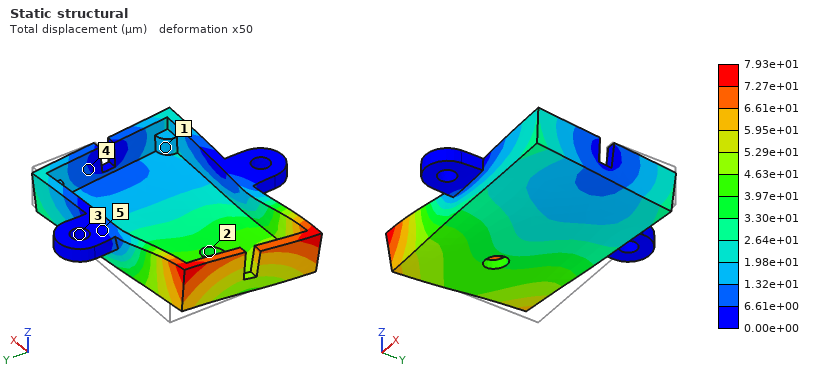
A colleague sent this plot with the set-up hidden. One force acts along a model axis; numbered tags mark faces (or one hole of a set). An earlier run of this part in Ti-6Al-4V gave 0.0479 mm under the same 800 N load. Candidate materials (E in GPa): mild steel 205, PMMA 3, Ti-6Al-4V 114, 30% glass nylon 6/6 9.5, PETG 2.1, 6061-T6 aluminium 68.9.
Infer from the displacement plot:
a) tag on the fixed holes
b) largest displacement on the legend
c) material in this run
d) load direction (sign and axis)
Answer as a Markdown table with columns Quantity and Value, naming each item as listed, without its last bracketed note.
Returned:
| Quantity | Value |
|---|---|
| tag on the fixed holes | 3 |
| largest displacement on the legend | 7.93e+01 µm |
| material in this run | 6061-T6 aluminium |
| load direction | -Y |
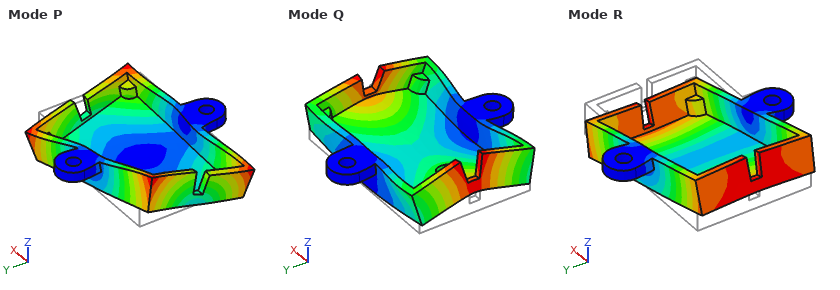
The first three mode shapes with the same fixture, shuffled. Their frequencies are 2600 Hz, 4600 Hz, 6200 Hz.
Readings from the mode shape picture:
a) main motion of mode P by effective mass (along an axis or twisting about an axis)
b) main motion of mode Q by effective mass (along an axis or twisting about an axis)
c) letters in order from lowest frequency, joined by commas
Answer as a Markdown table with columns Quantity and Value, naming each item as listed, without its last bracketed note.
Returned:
| Quantity | Value |
|---|---|
| main motion of mode P by effective mass | twisting about Z |
| main motion of mode Q by effective mass | along Z |
| letters in order from lowest frequency, joined by commas | R, P, Q |
